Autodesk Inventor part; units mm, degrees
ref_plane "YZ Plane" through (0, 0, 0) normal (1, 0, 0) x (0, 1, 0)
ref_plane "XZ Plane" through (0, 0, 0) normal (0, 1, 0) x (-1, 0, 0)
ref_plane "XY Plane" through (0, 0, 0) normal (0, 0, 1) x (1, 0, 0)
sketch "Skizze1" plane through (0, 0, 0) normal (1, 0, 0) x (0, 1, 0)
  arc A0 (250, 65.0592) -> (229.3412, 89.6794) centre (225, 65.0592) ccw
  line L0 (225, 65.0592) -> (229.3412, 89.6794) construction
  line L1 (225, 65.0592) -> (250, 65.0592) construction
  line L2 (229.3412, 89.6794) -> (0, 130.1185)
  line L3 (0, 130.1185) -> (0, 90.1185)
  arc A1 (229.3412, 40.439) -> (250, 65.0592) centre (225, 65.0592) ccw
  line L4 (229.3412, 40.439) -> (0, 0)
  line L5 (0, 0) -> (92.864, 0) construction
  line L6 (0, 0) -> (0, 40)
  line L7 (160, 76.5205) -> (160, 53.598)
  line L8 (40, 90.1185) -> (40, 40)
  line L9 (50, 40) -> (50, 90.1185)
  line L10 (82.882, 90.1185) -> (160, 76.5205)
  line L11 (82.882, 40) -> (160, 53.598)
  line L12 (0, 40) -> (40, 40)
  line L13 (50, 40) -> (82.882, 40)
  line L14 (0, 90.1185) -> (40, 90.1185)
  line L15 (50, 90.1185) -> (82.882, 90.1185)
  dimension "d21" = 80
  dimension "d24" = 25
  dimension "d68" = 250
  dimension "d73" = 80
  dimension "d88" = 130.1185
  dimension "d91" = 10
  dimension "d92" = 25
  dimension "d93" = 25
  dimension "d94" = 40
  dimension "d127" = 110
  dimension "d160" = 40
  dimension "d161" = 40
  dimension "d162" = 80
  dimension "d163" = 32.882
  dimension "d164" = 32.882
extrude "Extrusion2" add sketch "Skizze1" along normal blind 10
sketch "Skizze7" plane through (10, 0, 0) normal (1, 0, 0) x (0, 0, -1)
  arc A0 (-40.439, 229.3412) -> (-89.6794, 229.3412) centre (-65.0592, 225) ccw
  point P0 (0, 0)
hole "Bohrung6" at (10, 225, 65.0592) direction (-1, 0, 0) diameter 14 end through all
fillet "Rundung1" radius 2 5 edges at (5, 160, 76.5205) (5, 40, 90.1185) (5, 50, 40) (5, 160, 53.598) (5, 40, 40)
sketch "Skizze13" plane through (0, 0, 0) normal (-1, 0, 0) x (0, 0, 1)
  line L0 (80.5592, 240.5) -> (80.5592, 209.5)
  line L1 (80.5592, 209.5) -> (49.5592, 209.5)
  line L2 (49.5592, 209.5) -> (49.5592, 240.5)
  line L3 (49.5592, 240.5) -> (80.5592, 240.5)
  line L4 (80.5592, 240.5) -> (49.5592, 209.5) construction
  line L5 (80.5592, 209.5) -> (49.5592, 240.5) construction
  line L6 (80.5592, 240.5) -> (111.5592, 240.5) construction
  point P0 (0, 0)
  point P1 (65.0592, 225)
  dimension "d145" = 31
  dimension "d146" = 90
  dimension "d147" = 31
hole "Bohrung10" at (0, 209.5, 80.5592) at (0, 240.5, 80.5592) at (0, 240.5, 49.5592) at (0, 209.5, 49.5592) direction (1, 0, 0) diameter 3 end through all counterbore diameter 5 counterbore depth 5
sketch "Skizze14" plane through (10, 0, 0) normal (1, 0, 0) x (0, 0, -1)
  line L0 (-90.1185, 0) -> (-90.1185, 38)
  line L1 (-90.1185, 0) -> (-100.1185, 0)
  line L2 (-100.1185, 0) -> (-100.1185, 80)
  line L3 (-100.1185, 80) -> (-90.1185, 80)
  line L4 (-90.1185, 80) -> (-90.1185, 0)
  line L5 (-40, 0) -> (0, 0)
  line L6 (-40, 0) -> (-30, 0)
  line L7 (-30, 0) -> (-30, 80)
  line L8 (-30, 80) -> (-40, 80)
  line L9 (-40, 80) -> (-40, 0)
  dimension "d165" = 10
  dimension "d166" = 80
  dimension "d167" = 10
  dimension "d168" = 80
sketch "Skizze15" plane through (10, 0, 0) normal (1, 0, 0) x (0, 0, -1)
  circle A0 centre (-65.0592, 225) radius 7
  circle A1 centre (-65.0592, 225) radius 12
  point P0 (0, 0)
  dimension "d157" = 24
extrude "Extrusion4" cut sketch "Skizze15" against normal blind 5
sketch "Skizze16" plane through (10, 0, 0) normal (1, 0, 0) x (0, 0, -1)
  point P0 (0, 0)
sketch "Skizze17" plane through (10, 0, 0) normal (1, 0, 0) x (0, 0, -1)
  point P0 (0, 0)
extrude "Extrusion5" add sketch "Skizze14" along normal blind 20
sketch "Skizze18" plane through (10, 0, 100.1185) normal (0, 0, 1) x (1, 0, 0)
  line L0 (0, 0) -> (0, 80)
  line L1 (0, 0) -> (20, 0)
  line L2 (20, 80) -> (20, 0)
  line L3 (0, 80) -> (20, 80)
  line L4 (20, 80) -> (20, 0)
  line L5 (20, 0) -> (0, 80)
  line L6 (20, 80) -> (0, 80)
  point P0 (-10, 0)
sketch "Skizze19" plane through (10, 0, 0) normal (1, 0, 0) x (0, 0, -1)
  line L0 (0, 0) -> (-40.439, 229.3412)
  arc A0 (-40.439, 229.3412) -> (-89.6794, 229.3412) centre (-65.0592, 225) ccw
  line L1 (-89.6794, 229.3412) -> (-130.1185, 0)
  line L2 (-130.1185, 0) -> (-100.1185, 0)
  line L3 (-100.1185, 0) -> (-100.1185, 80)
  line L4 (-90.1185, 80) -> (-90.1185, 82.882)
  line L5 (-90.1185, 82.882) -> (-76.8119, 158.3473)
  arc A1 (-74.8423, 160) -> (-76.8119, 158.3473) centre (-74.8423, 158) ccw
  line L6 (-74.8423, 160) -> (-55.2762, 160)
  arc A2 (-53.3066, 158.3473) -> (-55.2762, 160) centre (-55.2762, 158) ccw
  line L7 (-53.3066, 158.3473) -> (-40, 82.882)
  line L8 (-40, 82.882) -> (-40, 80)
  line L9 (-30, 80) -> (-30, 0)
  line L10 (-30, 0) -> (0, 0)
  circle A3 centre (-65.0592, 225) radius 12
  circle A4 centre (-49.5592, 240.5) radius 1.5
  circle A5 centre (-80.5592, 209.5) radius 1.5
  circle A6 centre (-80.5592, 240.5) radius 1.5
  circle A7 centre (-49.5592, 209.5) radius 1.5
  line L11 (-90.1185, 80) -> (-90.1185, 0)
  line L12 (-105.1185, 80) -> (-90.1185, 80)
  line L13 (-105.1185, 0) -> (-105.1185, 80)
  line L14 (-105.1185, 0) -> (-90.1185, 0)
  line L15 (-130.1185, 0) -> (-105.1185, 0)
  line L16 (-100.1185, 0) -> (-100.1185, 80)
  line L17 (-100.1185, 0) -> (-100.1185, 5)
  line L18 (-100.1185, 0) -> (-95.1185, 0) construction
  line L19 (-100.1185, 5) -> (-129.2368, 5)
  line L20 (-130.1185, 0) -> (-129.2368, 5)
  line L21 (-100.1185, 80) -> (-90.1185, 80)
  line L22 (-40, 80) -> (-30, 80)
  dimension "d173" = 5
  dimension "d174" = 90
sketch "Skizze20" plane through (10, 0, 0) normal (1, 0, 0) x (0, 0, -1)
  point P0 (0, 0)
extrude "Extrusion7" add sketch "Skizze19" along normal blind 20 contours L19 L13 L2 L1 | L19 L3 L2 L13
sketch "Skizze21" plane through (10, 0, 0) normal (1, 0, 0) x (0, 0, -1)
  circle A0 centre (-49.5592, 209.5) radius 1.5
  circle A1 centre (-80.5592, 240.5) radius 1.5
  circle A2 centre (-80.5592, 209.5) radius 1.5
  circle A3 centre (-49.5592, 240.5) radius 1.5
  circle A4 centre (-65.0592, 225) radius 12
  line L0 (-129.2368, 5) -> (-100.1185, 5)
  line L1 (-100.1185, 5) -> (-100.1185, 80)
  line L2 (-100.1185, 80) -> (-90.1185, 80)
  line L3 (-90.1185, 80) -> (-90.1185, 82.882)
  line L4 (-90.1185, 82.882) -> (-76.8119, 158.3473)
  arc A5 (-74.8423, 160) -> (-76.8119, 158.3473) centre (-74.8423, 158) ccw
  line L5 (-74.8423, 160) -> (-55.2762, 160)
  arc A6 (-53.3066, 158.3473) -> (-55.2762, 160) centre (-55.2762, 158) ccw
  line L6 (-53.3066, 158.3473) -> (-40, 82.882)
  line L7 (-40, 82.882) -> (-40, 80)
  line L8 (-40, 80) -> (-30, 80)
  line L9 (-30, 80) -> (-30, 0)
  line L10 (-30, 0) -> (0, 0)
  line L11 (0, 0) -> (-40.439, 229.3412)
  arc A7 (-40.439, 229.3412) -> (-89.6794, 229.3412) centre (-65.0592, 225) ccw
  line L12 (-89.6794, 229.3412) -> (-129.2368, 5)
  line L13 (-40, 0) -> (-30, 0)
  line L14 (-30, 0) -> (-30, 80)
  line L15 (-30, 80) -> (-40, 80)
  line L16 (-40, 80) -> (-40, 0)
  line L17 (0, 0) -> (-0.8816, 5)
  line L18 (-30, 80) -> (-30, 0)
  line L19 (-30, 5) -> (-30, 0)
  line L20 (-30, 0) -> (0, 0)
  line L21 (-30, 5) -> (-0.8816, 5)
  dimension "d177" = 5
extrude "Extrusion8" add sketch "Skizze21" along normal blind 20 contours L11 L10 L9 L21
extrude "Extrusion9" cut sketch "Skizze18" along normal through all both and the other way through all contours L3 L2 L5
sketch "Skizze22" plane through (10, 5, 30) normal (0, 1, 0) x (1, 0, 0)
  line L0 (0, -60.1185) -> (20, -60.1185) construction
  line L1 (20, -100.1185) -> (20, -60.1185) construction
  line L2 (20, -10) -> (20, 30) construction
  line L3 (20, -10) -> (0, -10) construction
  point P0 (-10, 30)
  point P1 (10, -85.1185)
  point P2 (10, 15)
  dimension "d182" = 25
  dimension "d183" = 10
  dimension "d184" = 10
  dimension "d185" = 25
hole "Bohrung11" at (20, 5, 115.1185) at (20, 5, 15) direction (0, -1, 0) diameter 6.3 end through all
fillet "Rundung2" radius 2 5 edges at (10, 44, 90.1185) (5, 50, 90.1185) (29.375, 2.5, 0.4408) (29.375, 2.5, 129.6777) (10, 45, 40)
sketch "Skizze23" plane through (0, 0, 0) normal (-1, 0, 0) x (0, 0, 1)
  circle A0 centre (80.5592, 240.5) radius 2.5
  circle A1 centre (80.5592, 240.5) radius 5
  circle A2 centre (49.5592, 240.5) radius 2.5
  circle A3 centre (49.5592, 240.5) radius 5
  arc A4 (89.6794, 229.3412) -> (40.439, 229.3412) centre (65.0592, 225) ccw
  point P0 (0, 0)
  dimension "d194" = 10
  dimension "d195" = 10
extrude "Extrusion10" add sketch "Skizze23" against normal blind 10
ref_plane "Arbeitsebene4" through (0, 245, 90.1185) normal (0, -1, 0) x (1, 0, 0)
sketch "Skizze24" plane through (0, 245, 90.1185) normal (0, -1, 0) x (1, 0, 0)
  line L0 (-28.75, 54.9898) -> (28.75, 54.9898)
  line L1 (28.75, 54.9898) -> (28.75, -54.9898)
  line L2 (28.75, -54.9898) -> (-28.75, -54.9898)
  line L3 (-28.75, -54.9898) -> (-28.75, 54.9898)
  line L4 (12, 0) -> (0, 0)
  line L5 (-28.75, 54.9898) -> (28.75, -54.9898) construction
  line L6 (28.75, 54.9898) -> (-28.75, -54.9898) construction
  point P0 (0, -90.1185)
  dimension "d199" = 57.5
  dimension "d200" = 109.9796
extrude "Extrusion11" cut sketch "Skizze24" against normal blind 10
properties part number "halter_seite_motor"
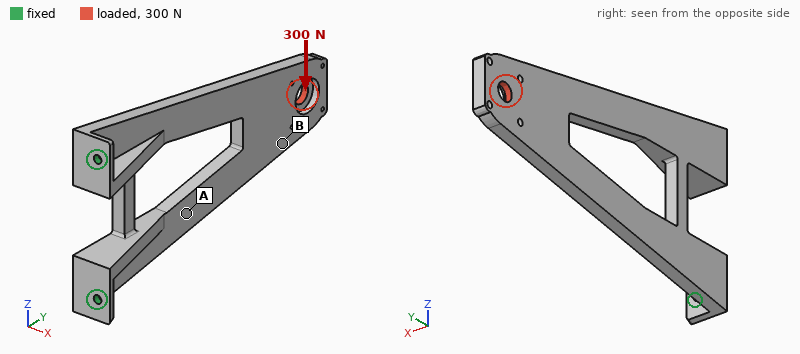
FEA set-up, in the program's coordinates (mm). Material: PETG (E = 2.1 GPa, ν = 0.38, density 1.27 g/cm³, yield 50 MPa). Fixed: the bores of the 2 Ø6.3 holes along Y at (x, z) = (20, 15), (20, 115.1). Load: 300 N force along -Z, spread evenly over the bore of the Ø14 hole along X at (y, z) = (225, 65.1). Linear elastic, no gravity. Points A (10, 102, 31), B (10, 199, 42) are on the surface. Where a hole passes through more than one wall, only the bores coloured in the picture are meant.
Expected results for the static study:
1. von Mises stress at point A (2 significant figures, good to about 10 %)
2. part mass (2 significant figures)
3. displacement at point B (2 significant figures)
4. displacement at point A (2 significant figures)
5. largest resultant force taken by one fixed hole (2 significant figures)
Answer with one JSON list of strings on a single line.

["4.6 MPa", "210 g", "2.7 mm", "1.8 mm", "670 N"]
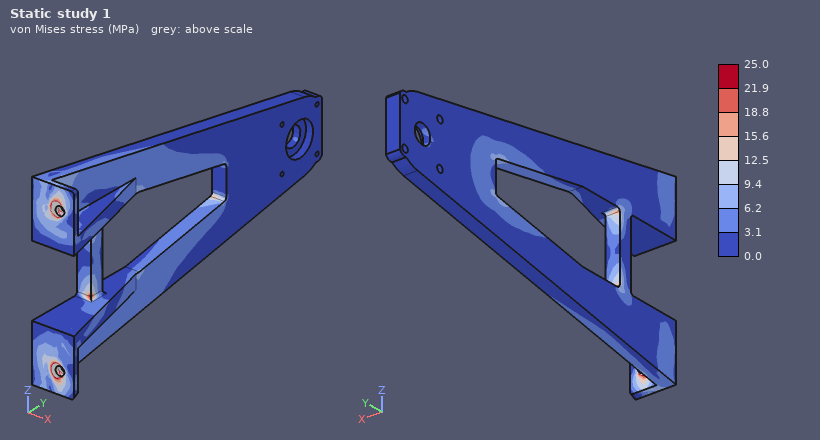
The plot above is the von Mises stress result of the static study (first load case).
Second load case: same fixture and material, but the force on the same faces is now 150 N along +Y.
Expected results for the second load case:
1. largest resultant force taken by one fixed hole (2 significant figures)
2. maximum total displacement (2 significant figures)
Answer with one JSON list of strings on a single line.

["76 N", "3.1 mm"]
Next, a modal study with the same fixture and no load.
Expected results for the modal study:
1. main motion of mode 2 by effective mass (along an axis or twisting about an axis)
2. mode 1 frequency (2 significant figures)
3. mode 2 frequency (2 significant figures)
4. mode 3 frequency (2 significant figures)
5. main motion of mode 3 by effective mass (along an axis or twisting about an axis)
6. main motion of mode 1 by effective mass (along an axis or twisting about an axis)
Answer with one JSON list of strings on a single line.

["along Z", "34 Hz", "160 Hz", "190 Hz", "along X", "along X"]
